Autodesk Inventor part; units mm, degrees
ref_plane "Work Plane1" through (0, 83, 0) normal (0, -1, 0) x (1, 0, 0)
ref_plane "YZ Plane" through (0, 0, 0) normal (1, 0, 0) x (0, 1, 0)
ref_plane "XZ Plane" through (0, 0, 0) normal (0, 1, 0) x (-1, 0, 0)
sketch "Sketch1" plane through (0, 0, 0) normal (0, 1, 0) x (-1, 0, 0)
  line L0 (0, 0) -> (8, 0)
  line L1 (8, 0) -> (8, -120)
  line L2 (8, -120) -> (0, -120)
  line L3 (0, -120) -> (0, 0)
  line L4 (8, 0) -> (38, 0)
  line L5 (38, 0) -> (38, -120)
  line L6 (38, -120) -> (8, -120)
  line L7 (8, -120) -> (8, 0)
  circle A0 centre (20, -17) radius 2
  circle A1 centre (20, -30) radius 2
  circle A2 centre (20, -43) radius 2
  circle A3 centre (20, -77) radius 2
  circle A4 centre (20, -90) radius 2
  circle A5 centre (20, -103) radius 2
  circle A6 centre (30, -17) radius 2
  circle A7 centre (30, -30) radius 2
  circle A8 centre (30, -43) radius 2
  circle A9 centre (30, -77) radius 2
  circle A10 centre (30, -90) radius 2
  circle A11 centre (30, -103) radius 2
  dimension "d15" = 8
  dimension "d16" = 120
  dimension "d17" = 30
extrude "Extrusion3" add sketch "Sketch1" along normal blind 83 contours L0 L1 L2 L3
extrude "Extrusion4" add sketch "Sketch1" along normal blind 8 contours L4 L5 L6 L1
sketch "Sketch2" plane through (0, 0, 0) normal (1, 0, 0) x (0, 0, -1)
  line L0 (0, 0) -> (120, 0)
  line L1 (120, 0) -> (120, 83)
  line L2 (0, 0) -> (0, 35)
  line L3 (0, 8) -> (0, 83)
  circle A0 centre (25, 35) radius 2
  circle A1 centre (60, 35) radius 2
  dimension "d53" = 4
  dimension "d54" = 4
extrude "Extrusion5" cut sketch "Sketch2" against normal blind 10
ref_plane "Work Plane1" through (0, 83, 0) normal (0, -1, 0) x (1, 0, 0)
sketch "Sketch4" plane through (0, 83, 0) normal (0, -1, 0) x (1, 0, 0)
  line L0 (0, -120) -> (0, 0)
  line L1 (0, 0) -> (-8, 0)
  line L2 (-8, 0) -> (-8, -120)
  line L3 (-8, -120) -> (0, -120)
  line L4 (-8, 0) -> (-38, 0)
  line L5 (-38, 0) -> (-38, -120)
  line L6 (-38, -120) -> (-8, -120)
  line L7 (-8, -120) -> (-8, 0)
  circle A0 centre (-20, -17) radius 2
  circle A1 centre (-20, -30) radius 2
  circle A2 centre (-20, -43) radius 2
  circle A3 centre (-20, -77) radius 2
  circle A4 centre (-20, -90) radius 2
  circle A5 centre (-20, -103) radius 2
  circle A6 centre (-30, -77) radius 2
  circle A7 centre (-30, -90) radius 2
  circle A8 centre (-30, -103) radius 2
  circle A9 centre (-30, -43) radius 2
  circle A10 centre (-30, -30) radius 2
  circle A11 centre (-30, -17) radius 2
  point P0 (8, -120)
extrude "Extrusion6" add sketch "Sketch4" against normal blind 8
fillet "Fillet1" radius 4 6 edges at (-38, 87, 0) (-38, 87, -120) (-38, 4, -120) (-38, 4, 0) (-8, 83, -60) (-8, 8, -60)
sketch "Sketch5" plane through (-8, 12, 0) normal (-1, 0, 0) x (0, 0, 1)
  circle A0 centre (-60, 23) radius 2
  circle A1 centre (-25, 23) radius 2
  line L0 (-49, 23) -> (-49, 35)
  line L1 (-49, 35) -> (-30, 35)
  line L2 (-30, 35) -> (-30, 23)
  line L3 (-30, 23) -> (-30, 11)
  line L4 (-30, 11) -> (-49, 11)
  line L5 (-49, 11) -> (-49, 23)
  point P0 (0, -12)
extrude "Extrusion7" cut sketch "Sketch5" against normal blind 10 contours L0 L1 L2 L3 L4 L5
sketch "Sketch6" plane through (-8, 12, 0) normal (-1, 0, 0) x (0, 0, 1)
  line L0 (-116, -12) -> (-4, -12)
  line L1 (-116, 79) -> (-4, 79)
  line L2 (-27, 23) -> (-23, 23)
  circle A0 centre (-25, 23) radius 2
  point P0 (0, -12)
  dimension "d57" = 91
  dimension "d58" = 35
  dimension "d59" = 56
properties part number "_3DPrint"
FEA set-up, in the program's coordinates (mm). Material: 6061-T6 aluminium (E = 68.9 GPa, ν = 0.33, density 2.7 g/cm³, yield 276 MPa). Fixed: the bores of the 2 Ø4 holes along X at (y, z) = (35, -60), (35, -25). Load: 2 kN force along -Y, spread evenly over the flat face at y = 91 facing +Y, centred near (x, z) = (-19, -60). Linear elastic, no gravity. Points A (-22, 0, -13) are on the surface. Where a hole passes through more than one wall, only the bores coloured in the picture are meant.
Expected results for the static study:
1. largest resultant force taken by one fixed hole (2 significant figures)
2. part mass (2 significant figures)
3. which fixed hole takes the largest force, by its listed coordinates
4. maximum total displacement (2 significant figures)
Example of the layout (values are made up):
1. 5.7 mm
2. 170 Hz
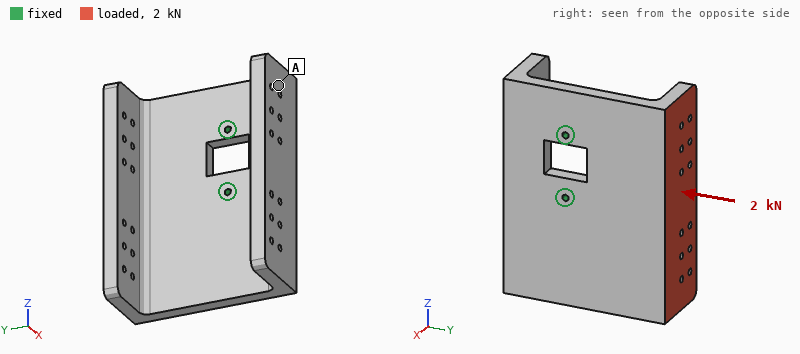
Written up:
1. 1.9 kN
2. 380 g
3. (35, -60)
4. 0.30 mm
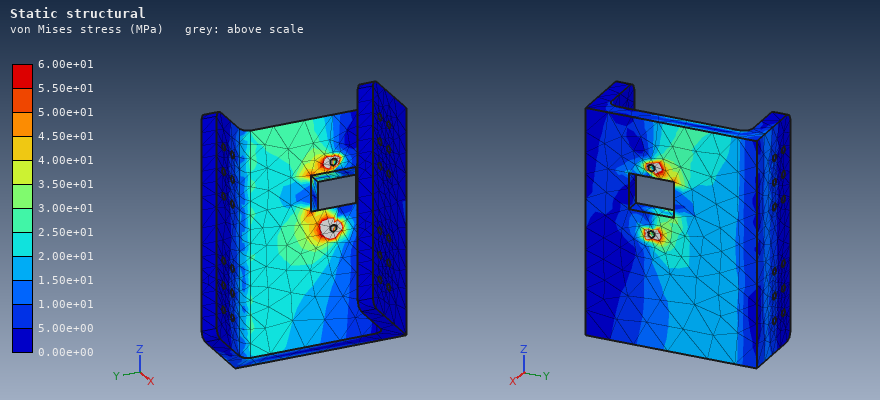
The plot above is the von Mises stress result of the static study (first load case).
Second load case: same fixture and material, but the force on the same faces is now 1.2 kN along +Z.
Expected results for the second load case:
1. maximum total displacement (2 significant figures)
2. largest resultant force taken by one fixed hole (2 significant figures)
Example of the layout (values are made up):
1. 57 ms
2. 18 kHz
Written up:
1. 99 µm
2. 1.9 kN
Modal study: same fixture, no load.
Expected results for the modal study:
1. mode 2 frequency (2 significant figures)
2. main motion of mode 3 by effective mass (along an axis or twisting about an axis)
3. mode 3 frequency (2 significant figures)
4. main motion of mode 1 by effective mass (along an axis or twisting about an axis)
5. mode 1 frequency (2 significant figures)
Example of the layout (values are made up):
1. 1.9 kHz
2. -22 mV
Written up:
1. 1300 Hz
2. along X
3. 1500 Hz
4. along X
5. 780 Hz
